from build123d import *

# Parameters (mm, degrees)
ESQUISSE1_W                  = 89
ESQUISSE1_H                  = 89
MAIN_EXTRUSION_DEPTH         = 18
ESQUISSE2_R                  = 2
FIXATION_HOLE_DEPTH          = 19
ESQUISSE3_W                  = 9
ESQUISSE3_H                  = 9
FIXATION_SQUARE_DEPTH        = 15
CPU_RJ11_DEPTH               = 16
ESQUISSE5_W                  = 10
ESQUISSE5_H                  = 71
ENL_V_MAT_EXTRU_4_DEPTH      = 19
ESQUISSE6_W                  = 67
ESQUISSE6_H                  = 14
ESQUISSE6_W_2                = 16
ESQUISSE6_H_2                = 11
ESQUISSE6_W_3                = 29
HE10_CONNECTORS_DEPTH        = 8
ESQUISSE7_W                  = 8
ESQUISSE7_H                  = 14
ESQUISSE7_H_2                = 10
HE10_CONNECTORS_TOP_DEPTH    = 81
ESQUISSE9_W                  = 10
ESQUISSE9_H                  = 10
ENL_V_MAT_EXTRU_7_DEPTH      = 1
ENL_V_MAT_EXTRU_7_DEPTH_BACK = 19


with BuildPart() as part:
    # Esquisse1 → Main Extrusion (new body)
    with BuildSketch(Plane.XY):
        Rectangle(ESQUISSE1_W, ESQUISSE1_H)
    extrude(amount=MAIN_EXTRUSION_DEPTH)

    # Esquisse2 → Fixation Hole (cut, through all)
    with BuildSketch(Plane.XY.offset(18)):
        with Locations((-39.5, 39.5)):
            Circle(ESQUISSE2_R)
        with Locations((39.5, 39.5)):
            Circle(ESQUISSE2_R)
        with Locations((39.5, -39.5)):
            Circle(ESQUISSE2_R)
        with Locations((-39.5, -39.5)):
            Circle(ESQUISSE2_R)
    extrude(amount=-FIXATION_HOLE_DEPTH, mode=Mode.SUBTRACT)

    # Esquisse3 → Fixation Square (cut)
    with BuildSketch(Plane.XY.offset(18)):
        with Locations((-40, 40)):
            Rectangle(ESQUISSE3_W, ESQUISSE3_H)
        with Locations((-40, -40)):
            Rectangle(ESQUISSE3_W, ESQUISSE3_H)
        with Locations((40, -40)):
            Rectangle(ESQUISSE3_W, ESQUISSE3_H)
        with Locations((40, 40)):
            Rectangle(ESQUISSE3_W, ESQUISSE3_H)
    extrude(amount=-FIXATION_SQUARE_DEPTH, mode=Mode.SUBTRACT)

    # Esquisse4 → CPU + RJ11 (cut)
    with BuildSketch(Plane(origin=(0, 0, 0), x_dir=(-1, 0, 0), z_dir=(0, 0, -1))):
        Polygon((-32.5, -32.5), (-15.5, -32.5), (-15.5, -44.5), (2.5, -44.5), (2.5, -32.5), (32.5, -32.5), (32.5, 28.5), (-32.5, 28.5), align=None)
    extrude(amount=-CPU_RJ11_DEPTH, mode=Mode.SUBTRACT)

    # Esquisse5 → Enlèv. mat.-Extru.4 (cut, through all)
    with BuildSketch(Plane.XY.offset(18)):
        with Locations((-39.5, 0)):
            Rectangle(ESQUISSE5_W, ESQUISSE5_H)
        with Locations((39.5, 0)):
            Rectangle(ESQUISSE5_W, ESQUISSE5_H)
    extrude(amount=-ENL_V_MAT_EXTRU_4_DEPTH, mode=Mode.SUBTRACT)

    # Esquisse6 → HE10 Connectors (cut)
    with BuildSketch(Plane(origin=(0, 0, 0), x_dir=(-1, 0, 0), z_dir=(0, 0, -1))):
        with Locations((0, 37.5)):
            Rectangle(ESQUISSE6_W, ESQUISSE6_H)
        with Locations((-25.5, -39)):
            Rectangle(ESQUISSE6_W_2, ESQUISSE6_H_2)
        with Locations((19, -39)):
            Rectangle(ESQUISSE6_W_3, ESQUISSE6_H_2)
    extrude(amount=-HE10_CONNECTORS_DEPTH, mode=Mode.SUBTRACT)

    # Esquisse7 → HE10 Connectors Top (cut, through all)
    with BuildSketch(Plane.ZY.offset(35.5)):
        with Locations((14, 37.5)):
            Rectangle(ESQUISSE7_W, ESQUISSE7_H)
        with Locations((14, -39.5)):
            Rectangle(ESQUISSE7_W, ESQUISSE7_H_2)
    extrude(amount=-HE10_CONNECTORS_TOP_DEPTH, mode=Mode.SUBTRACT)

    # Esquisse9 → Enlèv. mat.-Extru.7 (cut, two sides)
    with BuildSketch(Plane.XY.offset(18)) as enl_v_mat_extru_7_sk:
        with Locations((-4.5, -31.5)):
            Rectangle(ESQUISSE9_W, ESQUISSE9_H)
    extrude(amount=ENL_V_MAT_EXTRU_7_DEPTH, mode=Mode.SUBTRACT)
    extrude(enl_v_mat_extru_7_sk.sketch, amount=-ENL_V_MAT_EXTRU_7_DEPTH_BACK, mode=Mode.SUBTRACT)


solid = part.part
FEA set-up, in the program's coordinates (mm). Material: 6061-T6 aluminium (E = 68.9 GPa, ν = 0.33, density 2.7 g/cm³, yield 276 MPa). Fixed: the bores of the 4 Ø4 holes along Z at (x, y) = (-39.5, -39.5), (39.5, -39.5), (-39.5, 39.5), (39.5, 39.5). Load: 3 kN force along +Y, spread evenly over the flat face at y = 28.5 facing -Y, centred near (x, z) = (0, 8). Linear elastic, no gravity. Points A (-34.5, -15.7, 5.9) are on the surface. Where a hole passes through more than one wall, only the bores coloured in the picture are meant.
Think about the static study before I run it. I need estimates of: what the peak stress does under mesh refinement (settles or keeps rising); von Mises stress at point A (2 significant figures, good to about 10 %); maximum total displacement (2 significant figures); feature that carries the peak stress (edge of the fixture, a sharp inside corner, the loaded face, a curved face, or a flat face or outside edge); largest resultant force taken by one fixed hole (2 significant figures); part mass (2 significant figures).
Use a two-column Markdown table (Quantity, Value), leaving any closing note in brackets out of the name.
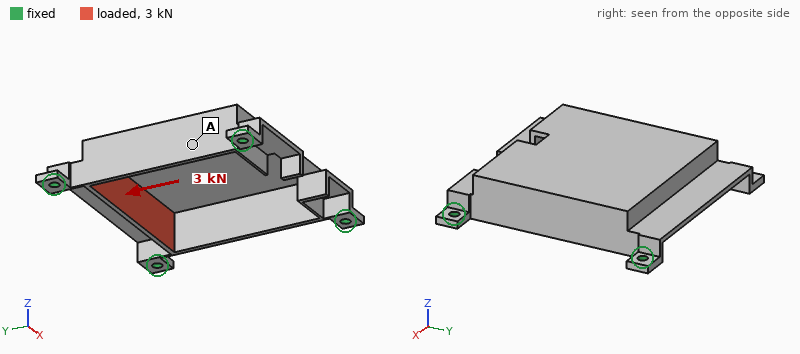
| Quantity | Value |
|---|---|
| what the peak stress does under mesh refinement | keeps rising |
| von Mises stress at point A | 22 MPa |
| maximum total displacement | 0.33 mm |
| feature that carries the peak stress | edge of the fixture |
| largest resultant force taken by one fixed hole | 940 N |
| part mass | 56 g |
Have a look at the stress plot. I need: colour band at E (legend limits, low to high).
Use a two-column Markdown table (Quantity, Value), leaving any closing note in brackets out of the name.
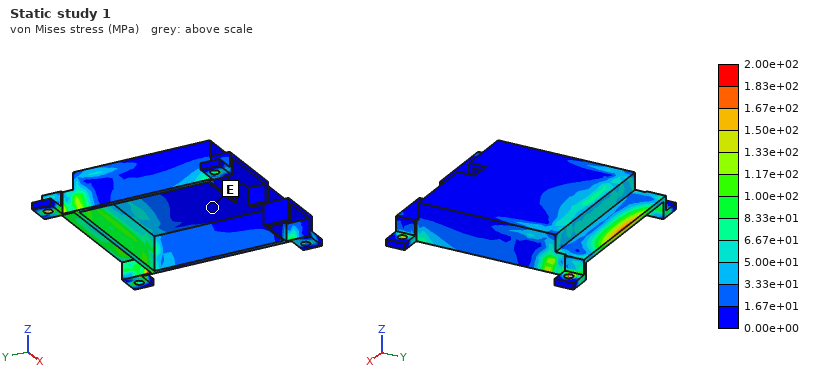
| Quantity | Value |
|---|---|
| colour band at E | 0.00e+00 to 1.67e+01 MPa |
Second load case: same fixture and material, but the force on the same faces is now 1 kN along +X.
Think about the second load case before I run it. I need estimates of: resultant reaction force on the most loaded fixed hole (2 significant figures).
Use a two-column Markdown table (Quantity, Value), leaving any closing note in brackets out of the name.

| Quantity | Value |
|---|---|
| resultant reaction force on the most loaded fixed hole | 400 N |
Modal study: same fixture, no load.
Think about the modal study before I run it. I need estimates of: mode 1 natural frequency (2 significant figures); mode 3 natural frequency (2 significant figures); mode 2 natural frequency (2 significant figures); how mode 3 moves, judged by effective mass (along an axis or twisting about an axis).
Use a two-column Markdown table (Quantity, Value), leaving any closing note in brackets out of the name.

| Quantity | Value |
|---|---|
| mode 1 natural frequency | 2700 Hz |
| mode 3 natural frequency | 3300 Hz |
| mode 2 natural frequency | 2800 Hz |
| how mode 3 moves, judged by effective mass | along X |
